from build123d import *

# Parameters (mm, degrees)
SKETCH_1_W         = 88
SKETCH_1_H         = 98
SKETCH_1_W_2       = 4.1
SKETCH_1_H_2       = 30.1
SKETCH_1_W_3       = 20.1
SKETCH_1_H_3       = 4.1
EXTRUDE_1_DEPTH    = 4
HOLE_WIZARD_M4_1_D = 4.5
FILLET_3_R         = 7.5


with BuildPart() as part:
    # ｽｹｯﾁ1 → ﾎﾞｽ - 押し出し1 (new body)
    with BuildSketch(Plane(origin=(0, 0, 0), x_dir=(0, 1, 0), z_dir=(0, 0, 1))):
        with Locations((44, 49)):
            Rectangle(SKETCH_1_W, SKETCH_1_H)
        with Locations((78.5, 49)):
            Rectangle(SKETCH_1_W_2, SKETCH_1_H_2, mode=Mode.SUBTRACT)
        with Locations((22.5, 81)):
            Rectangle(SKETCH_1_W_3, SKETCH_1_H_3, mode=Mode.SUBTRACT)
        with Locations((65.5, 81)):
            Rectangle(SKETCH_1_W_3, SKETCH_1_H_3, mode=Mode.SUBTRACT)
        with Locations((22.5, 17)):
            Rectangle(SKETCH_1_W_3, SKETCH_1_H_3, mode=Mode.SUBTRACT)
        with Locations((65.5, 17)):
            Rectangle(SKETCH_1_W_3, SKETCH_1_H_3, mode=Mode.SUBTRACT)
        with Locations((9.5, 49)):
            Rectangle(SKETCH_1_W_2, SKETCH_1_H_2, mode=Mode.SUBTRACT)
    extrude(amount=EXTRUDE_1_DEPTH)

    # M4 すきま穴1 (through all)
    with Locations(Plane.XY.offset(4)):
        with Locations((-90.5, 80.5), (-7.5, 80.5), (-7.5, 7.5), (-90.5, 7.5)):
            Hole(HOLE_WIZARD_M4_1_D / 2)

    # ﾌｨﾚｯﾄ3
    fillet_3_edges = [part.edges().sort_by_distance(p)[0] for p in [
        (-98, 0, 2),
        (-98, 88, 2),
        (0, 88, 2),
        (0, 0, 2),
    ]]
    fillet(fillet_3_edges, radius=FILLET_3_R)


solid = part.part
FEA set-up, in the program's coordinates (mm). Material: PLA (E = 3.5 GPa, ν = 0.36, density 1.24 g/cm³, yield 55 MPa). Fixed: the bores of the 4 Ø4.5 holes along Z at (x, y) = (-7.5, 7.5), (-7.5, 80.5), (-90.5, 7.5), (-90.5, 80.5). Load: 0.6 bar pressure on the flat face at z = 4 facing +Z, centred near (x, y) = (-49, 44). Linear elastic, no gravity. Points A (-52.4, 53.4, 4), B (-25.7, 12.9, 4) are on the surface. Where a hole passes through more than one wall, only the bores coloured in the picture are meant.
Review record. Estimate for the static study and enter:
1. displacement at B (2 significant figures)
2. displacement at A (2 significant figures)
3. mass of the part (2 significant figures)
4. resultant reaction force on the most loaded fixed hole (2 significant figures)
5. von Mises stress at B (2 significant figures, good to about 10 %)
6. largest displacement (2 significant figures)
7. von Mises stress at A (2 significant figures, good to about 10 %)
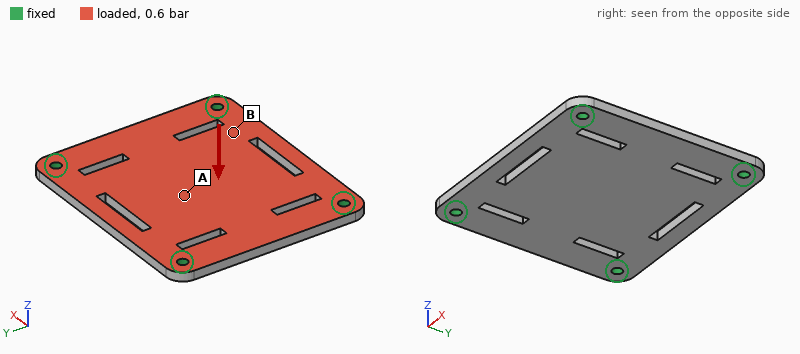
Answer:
0.37 mm
0.83 mm
39 g
120 N
3.0 MPa
0.86 mm
7.5 MPa
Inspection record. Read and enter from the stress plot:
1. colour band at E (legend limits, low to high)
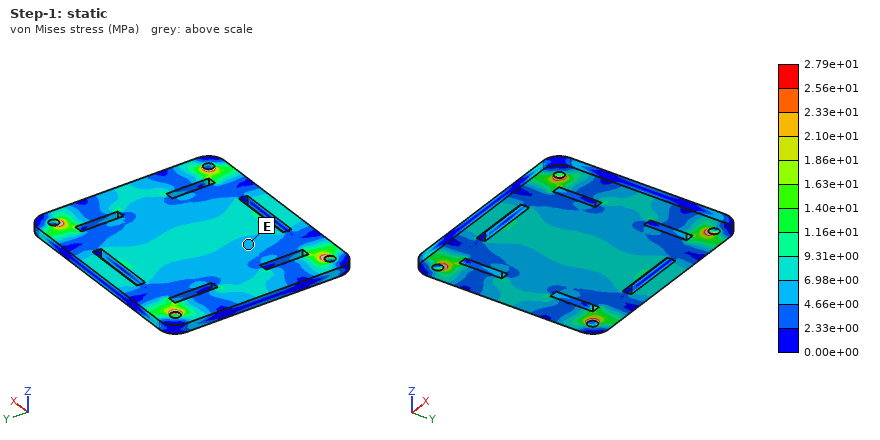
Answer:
4.66e+00 to 6.98e+00 MPa
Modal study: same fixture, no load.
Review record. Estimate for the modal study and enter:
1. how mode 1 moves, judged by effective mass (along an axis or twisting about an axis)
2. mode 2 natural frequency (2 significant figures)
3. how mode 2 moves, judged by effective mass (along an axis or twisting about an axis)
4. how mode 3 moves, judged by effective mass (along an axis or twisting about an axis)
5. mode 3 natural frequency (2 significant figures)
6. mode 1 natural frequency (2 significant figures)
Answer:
along Z
1100 Hz
twisting about X
twisting about Y
1300 Hz
710 Hz
